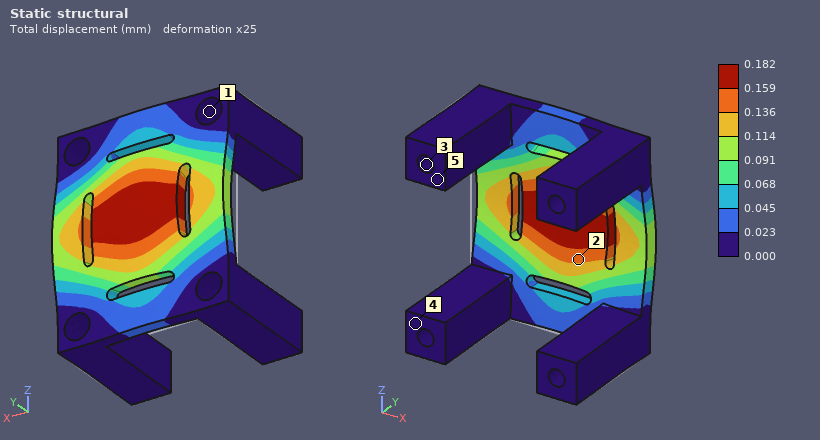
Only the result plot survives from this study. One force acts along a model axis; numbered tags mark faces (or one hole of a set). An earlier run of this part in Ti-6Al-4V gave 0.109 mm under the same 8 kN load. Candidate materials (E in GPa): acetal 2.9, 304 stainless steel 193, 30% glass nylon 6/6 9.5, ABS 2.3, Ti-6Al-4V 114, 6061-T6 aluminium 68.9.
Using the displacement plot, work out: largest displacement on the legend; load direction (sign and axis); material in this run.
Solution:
0.182 mm
+Y
6061-T6 aluminium
